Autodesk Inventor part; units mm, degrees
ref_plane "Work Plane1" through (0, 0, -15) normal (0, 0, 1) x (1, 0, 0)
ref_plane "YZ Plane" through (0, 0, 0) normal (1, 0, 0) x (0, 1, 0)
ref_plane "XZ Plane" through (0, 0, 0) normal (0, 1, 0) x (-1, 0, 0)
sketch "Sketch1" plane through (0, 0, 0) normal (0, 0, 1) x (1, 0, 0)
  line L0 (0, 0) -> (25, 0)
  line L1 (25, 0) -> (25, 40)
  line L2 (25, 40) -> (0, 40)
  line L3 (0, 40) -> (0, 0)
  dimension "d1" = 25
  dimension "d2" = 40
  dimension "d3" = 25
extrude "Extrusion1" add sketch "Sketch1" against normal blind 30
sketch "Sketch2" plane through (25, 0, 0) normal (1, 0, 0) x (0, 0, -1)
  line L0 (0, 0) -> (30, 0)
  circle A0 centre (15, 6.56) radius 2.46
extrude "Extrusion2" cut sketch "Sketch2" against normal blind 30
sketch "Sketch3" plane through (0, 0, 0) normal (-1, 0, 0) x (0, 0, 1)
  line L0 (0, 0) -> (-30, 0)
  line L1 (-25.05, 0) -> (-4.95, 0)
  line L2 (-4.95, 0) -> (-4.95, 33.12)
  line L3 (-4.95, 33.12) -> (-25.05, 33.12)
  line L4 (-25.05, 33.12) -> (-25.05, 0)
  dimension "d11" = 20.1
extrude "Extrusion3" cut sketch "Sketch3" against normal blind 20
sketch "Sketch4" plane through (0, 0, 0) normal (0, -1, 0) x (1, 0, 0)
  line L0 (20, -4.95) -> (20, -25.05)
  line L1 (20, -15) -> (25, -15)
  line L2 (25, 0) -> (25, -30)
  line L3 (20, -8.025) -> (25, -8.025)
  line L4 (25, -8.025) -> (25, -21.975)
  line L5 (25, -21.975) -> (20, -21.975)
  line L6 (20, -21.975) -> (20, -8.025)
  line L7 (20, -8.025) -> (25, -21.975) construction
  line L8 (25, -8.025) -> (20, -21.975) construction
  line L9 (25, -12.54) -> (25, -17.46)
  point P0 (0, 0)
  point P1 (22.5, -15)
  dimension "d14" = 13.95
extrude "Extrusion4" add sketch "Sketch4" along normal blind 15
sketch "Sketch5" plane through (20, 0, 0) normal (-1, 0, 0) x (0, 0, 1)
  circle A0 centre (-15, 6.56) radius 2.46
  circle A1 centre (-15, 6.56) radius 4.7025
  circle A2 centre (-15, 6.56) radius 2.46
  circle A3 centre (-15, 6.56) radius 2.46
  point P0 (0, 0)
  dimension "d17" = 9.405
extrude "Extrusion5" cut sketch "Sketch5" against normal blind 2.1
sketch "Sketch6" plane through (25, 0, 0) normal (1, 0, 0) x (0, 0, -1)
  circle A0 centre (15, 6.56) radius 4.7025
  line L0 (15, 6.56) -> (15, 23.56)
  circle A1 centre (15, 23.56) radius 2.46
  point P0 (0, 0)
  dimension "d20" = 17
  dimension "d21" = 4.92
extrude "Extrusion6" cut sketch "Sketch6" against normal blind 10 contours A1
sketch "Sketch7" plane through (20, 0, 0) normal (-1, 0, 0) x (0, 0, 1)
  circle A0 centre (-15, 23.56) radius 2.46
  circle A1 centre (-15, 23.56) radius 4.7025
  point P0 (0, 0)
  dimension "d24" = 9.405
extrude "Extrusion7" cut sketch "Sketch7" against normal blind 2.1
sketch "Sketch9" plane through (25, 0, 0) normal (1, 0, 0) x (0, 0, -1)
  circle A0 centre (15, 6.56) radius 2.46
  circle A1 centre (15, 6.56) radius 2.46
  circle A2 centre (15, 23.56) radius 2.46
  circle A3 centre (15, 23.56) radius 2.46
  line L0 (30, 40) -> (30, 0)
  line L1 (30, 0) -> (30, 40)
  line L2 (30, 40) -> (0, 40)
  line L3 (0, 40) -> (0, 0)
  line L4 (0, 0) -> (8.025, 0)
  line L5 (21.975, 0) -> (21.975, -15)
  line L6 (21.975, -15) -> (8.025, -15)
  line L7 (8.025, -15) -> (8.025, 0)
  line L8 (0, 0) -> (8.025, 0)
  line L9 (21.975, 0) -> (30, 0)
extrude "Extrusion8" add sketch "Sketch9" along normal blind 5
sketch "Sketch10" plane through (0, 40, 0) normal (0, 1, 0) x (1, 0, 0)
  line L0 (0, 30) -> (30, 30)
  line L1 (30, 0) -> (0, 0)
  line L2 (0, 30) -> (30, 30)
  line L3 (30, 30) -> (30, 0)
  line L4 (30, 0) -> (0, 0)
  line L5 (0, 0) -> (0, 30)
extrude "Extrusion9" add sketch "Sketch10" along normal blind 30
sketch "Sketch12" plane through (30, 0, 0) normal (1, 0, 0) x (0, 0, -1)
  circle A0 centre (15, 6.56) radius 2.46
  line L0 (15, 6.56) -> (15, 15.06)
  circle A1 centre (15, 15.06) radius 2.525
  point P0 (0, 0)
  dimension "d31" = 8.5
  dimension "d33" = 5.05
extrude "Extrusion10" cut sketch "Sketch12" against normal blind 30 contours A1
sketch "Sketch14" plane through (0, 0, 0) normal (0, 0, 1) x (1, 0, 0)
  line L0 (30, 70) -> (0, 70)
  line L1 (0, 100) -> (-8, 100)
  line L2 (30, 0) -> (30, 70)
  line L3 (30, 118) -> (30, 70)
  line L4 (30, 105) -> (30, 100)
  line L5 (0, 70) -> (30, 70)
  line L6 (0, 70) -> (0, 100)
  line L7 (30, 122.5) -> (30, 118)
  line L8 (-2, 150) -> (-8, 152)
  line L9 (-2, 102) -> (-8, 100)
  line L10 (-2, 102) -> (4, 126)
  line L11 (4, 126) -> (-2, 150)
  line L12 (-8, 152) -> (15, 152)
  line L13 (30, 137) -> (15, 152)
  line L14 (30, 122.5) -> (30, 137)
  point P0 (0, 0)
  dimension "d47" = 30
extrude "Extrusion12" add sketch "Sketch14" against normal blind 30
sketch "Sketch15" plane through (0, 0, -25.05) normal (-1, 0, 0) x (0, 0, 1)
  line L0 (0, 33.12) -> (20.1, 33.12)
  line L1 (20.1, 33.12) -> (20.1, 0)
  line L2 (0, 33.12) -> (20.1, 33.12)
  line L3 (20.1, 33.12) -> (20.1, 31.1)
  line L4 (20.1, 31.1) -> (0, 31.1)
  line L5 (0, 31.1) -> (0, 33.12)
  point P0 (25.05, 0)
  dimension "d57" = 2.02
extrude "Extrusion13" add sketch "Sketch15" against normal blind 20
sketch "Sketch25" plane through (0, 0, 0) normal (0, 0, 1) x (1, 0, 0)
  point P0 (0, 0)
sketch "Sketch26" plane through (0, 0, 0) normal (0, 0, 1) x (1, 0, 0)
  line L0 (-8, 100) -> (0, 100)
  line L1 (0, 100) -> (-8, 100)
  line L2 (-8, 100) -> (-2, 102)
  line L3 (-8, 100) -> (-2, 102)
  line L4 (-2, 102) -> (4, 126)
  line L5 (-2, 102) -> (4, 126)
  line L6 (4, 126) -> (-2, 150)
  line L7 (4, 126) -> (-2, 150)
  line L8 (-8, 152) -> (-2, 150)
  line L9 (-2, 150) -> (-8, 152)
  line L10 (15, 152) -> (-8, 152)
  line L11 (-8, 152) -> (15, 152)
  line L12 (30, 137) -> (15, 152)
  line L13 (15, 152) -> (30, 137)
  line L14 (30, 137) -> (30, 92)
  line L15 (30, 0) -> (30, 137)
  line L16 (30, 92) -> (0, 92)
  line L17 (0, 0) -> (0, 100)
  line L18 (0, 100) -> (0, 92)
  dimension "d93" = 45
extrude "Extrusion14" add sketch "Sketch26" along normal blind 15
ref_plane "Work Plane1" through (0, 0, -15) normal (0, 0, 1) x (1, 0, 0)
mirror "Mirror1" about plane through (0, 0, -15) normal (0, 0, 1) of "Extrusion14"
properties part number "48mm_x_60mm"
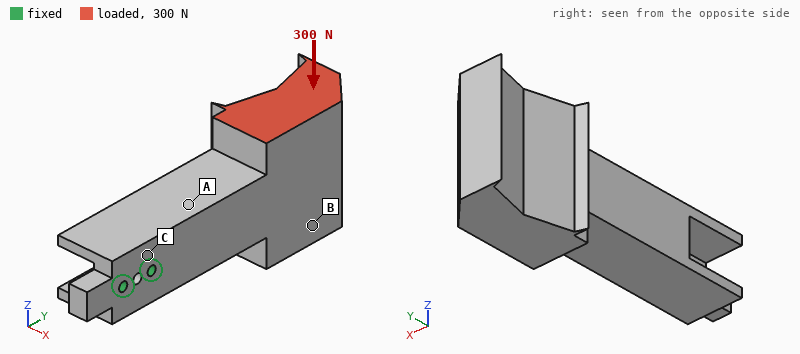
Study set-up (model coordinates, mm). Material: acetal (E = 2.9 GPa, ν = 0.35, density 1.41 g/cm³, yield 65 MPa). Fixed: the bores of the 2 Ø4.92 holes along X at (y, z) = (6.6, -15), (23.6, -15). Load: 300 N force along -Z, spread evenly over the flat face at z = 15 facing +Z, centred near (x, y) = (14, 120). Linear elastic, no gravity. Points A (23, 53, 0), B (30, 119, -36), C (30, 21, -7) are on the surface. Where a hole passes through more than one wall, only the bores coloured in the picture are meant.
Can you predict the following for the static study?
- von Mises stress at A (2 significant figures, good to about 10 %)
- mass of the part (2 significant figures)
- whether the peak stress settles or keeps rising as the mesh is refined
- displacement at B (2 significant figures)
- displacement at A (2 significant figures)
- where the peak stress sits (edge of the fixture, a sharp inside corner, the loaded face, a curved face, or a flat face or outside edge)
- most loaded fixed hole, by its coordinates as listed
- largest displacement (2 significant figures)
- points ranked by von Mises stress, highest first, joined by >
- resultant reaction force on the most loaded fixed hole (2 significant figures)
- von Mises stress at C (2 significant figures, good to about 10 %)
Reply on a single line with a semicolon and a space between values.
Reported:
5.0 MPa; 240 g; keeps rising; 1.4 mm; 0.41 mm; edge of the fixture; (23.6, -15); 2.0 mm; C > A > B; 1.6 kN; 9.6 MPa
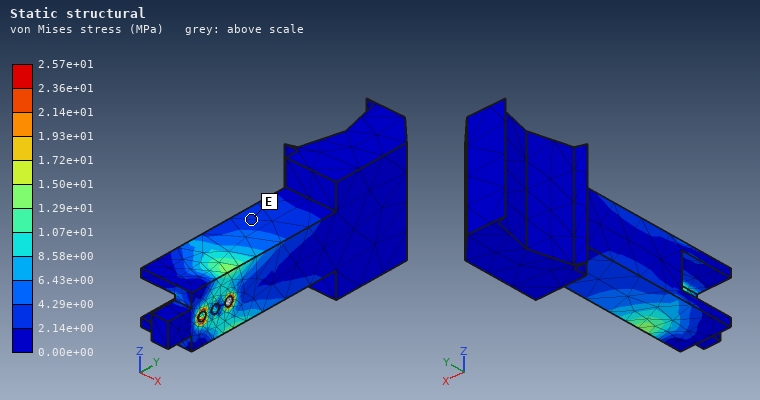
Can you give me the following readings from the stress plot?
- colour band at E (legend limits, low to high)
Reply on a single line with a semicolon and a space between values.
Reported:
2.14e+00 to 4.29e+00 MPa
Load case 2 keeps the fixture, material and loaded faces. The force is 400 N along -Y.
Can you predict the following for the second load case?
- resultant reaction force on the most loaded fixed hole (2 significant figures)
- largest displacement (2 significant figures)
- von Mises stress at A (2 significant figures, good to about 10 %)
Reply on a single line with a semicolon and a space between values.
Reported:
610 N; 1.1 mm; 3.4 MPa
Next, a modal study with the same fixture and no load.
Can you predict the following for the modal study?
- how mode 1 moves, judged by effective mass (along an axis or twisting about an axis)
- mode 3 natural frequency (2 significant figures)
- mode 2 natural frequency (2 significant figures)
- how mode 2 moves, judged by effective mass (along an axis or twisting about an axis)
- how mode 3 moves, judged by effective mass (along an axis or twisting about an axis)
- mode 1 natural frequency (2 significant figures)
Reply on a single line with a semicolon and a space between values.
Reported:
along X; 490 Hz; 180 Hz; along Z; twisting about Y; 160 Hz
